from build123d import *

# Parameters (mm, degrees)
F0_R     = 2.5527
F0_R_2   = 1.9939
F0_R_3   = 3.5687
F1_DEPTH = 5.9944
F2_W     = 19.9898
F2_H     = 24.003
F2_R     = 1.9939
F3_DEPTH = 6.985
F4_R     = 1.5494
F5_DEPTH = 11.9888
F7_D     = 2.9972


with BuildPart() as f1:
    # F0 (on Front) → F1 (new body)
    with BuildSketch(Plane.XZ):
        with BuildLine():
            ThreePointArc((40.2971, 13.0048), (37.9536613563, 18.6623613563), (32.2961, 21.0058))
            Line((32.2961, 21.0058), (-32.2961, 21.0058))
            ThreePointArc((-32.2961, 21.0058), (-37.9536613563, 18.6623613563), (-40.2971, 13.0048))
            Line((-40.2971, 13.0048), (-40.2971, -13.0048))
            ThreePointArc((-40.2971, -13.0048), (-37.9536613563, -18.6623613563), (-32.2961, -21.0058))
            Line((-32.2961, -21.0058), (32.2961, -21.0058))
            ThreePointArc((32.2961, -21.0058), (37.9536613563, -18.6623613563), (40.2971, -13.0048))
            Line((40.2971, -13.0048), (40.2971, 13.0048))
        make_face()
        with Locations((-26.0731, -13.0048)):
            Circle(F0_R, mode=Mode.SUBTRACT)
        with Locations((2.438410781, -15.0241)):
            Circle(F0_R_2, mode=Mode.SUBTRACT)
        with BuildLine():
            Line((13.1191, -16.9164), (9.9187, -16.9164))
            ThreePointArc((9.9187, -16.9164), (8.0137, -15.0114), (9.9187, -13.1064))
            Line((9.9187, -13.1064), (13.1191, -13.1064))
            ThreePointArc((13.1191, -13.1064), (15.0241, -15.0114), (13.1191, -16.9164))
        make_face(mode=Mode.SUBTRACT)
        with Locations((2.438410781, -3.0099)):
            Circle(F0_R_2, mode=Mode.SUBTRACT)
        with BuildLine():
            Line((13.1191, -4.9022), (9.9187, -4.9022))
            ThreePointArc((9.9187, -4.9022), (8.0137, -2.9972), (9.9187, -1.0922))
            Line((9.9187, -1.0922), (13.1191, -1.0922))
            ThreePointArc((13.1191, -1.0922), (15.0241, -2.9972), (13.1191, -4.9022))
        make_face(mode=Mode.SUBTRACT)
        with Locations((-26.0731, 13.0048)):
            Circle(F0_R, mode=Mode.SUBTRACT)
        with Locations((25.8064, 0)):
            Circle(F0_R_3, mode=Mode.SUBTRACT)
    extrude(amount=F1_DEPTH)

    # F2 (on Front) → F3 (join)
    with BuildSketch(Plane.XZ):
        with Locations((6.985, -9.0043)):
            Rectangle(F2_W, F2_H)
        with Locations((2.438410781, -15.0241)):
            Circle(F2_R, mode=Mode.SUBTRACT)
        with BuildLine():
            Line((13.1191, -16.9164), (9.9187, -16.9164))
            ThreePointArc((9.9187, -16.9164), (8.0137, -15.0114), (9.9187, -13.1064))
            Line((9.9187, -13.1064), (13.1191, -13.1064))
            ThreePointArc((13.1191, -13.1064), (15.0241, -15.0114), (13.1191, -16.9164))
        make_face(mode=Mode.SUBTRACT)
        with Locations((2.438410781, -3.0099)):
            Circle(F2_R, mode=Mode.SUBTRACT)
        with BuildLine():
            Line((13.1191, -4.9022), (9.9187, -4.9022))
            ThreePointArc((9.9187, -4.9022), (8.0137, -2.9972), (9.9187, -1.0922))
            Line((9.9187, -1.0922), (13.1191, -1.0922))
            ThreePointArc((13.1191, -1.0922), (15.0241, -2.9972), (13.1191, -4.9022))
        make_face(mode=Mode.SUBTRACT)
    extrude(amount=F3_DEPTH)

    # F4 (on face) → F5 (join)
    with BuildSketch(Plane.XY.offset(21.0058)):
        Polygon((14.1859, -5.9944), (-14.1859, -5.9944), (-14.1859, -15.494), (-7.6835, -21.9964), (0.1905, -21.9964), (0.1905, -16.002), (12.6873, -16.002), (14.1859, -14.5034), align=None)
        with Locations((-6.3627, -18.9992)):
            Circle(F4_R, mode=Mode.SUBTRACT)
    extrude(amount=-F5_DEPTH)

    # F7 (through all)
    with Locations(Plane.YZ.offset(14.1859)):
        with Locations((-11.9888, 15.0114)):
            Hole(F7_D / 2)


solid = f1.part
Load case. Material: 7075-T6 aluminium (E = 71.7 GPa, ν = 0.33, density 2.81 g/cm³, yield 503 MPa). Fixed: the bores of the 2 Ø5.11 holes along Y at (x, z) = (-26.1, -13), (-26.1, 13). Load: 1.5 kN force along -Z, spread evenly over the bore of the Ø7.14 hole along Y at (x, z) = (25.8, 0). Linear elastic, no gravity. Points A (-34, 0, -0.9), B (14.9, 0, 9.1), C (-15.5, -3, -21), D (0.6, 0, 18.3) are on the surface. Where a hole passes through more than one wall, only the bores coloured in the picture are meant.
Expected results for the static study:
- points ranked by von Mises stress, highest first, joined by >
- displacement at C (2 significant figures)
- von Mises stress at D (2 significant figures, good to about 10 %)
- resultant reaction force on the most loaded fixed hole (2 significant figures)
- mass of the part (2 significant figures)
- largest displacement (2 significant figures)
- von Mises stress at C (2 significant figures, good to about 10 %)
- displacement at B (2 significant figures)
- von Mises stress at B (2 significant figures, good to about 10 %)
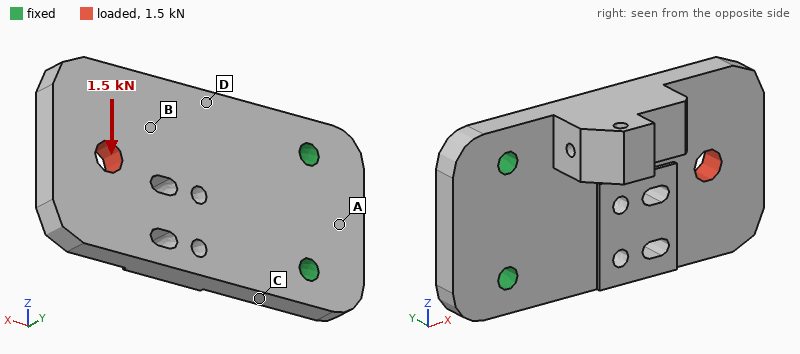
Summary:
C > D > B > A
10.0 µm
20 MPa
2.8 kN
66 g
59 µm
28 MPa
33 µm
13 MPa
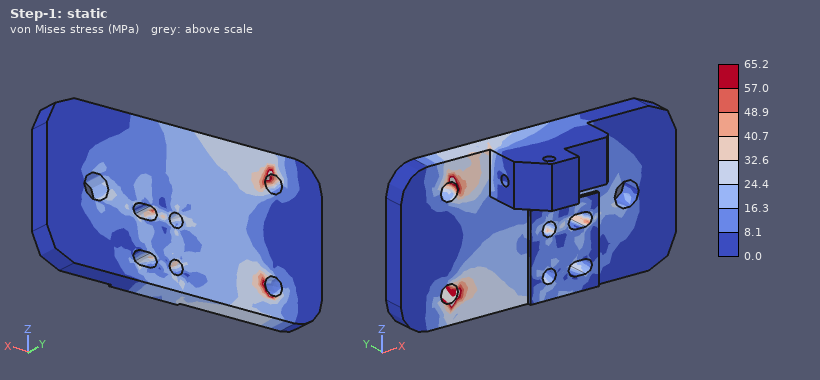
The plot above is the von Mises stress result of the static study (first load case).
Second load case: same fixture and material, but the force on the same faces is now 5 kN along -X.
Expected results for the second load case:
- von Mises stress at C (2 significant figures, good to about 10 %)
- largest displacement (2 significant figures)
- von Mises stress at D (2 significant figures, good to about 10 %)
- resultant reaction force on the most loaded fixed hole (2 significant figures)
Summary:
18 MPa
34 µm
19 MPa
2.5 kN
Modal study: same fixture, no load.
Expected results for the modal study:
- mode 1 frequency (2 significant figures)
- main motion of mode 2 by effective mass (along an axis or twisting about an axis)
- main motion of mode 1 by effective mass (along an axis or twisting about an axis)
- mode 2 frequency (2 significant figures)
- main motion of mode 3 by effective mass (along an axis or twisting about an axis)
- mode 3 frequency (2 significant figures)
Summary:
1200 Hz
twisting about X
along Y
3900 Hz
along Z
5800 Hz
